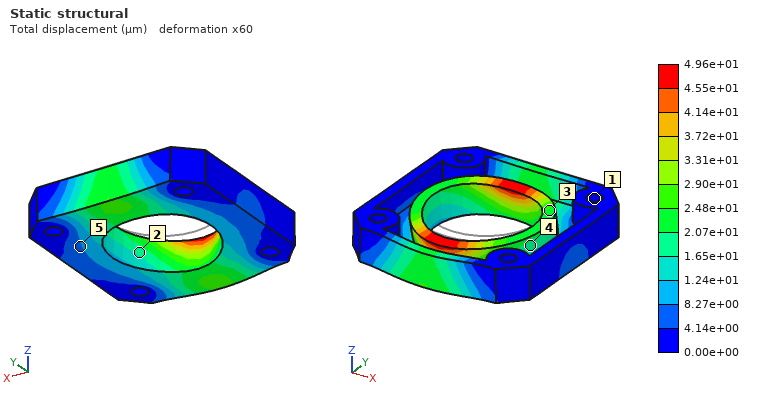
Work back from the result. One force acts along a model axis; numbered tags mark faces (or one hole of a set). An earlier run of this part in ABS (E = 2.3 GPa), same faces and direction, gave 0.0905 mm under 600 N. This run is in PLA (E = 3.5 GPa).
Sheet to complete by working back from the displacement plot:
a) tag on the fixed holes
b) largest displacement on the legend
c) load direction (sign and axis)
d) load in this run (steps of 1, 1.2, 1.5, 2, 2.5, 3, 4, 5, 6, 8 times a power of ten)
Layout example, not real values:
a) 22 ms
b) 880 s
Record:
a) 1
b) 4.96e+01 µm
c) -Y
d) 500 N
